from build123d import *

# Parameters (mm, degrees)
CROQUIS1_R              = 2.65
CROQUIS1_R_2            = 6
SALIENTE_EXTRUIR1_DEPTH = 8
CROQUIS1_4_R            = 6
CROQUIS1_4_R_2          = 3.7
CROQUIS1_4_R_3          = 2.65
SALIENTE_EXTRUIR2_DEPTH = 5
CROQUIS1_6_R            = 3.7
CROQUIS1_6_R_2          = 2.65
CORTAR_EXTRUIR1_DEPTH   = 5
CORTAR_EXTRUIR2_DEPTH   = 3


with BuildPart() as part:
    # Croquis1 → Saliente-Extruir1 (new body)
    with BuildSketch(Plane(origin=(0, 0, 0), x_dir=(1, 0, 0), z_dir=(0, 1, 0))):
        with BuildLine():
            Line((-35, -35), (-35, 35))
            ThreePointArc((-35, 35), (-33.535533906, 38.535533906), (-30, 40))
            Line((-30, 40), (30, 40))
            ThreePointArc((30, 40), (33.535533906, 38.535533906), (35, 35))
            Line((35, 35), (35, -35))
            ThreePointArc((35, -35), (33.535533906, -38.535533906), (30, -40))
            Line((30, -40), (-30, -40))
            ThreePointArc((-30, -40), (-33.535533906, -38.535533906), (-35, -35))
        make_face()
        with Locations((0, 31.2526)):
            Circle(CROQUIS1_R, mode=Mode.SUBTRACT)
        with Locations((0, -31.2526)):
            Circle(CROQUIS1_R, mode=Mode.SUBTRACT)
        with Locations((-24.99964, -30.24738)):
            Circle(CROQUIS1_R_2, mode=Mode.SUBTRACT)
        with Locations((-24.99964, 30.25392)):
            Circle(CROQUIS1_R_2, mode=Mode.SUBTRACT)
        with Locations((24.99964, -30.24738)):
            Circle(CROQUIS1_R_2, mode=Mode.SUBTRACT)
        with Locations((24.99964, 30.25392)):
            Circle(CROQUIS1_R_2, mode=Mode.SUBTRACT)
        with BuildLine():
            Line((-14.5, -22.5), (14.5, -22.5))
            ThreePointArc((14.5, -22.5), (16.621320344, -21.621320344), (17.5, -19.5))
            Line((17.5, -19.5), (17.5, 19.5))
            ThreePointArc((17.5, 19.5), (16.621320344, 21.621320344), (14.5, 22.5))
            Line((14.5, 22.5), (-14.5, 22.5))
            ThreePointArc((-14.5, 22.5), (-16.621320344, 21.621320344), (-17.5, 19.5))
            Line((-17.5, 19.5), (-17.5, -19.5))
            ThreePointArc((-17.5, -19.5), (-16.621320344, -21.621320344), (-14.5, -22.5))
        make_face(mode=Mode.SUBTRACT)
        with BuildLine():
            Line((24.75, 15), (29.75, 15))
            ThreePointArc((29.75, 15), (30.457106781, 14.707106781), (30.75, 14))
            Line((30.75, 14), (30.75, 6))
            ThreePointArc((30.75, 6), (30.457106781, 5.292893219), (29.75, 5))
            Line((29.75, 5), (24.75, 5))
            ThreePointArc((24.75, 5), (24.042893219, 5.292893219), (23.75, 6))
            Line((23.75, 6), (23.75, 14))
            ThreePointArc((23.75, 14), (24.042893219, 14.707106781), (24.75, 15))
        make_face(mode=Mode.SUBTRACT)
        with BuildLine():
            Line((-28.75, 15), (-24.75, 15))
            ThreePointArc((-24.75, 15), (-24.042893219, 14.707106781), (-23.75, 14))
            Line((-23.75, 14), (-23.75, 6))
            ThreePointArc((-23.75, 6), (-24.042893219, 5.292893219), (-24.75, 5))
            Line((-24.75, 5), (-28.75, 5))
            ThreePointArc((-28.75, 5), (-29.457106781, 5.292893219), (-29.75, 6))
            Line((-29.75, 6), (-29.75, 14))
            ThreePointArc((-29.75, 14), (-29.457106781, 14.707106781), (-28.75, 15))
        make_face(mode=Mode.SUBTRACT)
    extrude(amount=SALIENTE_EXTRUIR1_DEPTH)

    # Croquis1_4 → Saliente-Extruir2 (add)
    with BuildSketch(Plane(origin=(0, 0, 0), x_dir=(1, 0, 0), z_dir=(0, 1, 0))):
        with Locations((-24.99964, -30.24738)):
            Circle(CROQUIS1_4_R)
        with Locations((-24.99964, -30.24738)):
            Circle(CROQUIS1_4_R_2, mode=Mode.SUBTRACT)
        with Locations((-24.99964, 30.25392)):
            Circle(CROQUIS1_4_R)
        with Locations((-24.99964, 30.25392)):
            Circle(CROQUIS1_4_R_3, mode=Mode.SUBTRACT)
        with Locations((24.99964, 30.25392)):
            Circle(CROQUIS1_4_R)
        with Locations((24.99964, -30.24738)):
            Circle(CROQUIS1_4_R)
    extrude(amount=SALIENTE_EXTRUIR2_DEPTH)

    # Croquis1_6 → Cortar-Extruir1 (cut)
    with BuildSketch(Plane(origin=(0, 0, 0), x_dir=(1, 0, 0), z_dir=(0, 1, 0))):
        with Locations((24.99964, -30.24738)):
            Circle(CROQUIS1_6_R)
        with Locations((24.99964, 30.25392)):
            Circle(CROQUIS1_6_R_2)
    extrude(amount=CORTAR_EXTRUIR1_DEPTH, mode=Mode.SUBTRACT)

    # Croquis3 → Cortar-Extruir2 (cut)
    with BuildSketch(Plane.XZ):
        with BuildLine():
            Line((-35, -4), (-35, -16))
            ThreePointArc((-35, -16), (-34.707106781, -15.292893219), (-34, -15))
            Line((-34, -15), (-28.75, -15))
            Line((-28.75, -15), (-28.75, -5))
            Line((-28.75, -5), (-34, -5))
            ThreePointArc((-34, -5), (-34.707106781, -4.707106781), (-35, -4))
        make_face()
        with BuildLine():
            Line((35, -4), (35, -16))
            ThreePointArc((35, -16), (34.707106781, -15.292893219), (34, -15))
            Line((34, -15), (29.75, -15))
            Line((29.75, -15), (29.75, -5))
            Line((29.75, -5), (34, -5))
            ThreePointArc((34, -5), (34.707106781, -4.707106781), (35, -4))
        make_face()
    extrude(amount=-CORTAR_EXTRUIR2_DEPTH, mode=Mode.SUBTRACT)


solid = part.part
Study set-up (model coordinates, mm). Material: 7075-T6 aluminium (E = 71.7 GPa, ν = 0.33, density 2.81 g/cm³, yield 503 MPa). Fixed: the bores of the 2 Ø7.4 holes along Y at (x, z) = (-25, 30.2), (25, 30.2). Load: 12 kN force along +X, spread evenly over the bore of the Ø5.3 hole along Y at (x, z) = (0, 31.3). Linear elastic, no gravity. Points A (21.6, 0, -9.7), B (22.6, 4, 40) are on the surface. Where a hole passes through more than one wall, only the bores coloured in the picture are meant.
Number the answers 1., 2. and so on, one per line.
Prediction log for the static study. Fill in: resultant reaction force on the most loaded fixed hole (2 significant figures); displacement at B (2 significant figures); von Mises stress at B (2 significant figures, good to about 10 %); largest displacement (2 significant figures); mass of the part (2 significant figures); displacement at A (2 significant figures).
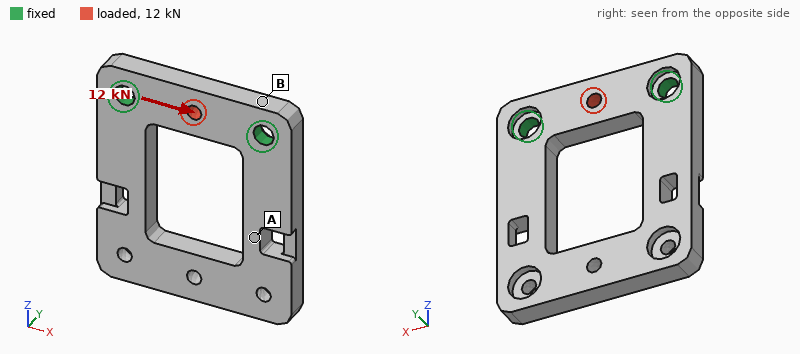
1. 6.0 kN
2. 6.1 µm
3. 22 MPa
4. 20 µm
5. 80 g
6. 7.2 µm
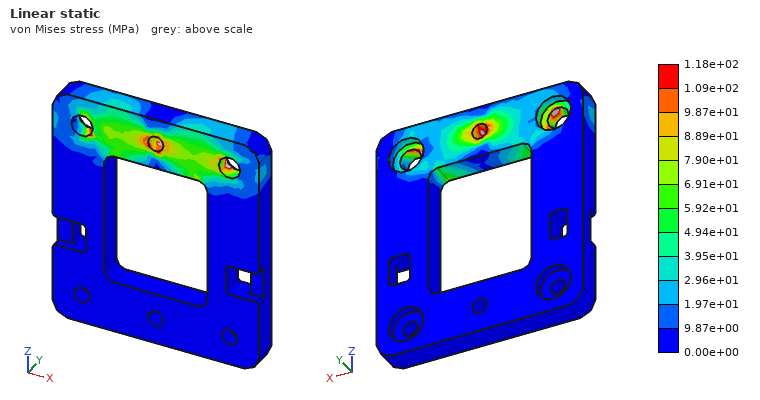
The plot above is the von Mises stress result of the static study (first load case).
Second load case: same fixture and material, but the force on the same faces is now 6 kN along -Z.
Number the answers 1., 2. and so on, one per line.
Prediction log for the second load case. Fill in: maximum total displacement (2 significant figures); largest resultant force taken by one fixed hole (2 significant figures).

1. 41 µm
2. 3.0 kN
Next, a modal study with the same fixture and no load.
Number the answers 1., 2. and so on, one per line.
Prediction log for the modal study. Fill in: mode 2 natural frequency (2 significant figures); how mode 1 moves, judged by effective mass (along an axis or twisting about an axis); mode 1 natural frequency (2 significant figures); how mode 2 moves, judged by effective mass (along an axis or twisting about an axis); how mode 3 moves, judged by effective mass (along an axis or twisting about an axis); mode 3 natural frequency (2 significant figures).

1. 2200 Hz
2. along Y
3. 970 Hz
4. twisting about Z
5. along X
6. 3300 Hz
